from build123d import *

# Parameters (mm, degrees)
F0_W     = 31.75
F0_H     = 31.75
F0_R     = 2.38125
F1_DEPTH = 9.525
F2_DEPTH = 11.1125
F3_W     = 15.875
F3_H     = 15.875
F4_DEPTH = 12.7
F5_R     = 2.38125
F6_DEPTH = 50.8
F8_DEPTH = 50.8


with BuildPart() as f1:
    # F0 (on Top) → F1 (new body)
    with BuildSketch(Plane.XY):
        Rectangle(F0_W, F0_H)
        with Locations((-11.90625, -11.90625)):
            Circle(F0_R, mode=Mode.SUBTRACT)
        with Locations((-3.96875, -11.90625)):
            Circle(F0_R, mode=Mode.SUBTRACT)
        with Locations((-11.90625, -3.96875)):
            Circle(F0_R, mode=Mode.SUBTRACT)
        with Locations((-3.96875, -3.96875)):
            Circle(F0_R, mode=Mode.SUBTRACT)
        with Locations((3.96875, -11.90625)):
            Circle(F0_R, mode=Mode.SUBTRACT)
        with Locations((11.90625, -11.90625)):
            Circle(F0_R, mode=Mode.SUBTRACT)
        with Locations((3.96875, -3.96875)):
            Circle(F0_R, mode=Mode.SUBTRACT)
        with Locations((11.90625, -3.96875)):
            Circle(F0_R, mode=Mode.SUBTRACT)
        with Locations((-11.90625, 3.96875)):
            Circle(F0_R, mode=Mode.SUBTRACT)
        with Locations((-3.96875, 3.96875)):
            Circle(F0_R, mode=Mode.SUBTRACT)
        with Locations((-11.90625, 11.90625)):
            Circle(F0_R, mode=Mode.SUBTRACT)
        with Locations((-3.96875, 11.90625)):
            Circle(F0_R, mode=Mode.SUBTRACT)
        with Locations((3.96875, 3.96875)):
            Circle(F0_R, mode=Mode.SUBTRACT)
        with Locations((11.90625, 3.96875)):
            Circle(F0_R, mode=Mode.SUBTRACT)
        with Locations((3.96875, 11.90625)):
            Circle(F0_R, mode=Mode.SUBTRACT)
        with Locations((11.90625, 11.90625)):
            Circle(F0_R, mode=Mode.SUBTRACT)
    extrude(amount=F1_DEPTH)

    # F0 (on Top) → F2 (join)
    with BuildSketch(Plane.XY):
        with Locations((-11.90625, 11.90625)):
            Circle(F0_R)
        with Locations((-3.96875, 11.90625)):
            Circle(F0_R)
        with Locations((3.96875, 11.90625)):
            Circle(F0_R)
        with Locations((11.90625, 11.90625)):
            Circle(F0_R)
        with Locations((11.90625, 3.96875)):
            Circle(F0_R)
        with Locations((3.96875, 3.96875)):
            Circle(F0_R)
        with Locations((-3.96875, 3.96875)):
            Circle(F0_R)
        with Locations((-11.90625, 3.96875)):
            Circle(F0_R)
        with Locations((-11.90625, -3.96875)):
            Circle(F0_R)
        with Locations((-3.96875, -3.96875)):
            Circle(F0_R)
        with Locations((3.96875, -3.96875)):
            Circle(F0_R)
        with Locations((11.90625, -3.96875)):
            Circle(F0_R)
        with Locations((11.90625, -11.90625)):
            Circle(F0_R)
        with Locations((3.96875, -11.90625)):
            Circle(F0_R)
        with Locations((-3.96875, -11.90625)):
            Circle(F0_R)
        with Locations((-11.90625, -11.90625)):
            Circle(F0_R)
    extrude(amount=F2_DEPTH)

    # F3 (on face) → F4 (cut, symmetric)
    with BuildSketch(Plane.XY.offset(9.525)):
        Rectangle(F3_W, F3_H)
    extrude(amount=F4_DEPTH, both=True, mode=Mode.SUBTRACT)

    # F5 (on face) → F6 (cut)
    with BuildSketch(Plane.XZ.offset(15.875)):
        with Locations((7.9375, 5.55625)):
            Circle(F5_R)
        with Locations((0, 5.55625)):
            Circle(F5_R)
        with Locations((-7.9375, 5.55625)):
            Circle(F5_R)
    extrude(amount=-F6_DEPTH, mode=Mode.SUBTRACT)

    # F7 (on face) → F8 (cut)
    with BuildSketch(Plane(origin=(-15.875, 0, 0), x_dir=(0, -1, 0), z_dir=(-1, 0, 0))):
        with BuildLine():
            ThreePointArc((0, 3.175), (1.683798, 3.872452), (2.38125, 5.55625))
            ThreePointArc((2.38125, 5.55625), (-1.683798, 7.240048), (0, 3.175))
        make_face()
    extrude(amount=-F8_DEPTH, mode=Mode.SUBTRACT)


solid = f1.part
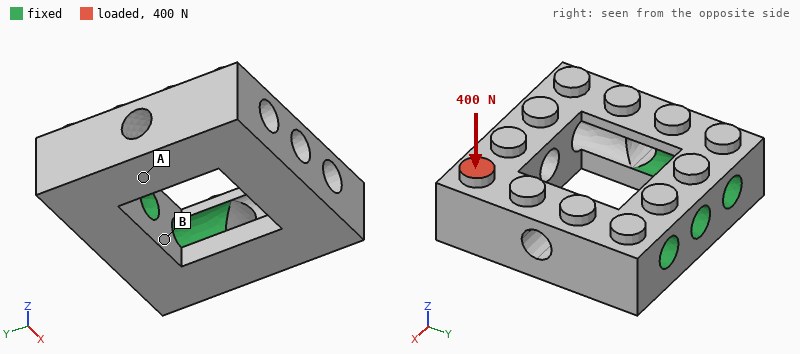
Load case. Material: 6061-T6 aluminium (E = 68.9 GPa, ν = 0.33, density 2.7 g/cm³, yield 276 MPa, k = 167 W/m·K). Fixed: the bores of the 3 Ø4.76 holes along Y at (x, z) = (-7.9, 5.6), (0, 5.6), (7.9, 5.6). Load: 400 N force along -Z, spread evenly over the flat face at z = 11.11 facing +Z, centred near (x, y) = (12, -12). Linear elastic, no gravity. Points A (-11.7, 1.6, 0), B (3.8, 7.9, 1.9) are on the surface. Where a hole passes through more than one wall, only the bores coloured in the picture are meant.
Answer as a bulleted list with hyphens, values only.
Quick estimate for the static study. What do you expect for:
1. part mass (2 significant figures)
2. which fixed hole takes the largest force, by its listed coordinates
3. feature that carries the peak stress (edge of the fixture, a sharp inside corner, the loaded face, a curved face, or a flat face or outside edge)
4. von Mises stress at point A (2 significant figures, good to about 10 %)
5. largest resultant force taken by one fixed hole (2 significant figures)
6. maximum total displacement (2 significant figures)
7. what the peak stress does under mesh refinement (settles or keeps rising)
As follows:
- 17 g
- (7.9, 5.6)
- edge of the fixture
- 14 MPa
- 360 N
- 32 µm
- keeps rising
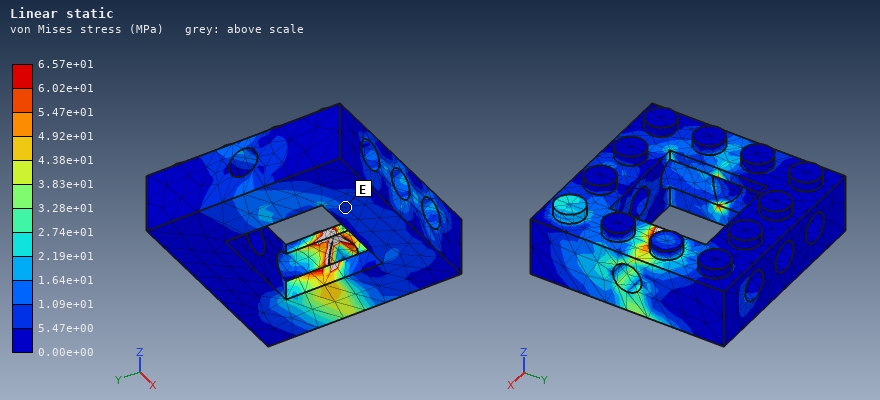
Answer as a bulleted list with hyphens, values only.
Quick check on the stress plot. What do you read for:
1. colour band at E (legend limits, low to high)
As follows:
- 5.47e+00 to 1.09e+01 MPa
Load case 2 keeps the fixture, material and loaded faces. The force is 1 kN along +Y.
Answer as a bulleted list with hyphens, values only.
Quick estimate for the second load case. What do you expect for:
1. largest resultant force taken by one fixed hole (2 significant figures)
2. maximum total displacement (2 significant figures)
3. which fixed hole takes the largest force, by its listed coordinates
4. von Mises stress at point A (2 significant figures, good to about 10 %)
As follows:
- 1.0 kN
- 45 µm
- (7.9, 5.6)
- 15 MPa
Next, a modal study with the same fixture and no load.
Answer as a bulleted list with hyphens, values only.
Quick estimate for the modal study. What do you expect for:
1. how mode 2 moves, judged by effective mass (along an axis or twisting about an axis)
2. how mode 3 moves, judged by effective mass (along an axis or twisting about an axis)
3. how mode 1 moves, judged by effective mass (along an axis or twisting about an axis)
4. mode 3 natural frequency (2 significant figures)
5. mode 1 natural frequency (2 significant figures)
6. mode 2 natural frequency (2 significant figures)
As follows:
- along X
- twisting about Y
- along Z
- 15 kHz
- 9800 Hz
- 14 kHz
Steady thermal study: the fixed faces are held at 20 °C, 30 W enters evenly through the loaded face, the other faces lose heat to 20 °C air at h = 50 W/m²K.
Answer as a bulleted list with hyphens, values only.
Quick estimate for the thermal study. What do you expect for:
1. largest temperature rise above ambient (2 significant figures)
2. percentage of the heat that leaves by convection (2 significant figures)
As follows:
- 65 K
- 7.4 %
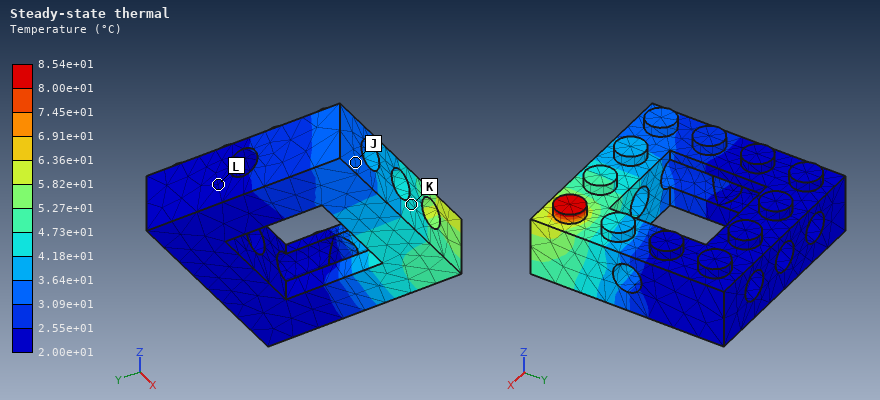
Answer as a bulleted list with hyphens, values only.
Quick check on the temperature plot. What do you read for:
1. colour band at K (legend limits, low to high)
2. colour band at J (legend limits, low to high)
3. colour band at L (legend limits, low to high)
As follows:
- 4.18e+01 to 4.73e+01 °C
- 3.09e+01 to 3.64e+01 °C
- 2.00e+01 to 2.55e+01 °C
